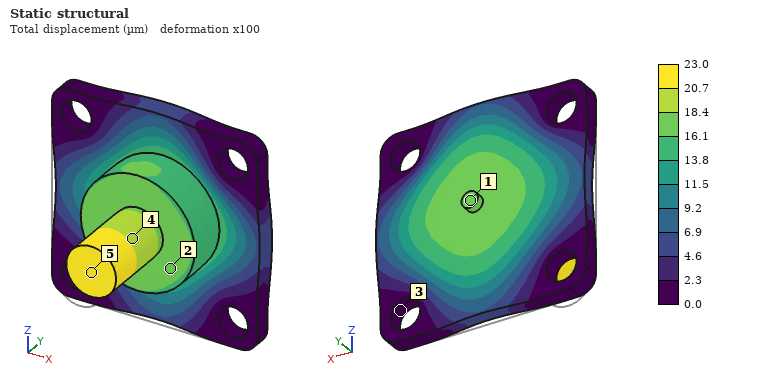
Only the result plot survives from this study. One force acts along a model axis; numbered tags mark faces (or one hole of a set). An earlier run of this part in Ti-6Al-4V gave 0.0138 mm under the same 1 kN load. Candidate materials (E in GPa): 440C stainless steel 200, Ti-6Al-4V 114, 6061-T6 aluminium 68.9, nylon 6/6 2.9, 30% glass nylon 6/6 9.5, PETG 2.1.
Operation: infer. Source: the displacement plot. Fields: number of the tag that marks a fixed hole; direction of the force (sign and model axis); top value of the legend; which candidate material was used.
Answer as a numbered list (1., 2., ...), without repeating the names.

1. 3
2. +Y
3. 23.0 µm
4. 6061-T6 aluminium
